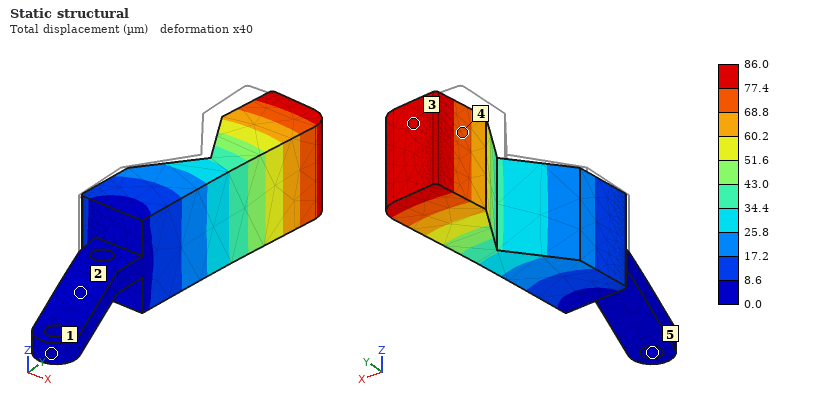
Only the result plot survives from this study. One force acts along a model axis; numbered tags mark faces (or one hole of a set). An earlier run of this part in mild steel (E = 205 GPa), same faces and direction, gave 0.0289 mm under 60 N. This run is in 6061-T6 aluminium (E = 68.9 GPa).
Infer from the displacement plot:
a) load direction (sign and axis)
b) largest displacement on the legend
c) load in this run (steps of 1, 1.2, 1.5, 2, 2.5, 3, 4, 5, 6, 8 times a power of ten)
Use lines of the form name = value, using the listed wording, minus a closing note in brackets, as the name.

load direction = +X
largest displacement on the legend = 86.0 µm
load in this run = 60 N
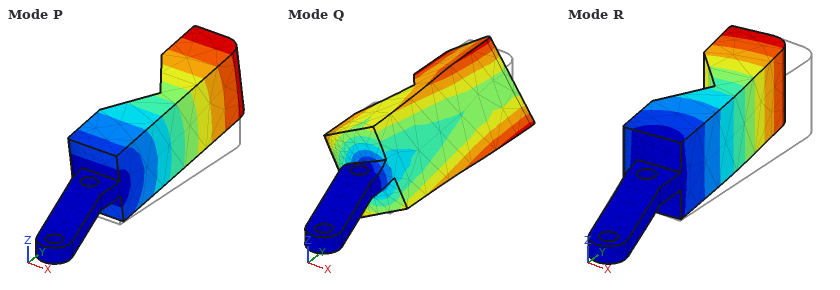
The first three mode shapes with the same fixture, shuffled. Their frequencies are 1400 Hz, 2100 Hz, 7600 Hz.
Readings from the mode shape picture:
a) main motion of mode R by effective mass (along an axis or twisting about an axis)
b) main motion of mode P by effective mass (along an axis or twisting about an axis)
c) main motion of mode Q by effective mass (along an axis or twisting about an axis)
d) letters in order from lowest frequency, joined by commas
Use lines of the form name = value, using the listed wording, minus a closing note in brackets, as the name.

main motion of mode R by effective mass = along X
main motion of mode P by effective mass = along Z
main motion of mode Q by effective mass = twisting about Y
letters in order from lowest frequency, joined by commas = P, R, Q
